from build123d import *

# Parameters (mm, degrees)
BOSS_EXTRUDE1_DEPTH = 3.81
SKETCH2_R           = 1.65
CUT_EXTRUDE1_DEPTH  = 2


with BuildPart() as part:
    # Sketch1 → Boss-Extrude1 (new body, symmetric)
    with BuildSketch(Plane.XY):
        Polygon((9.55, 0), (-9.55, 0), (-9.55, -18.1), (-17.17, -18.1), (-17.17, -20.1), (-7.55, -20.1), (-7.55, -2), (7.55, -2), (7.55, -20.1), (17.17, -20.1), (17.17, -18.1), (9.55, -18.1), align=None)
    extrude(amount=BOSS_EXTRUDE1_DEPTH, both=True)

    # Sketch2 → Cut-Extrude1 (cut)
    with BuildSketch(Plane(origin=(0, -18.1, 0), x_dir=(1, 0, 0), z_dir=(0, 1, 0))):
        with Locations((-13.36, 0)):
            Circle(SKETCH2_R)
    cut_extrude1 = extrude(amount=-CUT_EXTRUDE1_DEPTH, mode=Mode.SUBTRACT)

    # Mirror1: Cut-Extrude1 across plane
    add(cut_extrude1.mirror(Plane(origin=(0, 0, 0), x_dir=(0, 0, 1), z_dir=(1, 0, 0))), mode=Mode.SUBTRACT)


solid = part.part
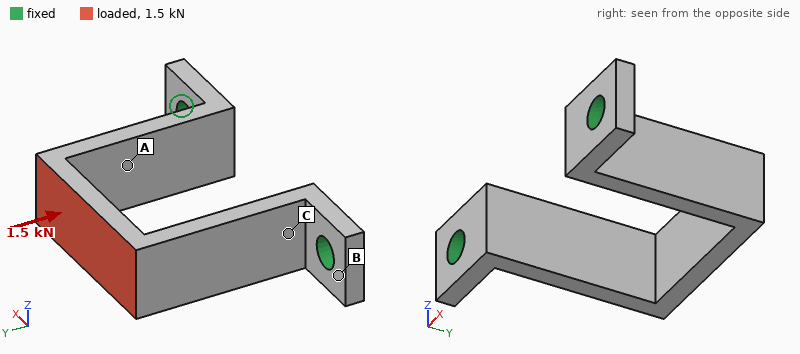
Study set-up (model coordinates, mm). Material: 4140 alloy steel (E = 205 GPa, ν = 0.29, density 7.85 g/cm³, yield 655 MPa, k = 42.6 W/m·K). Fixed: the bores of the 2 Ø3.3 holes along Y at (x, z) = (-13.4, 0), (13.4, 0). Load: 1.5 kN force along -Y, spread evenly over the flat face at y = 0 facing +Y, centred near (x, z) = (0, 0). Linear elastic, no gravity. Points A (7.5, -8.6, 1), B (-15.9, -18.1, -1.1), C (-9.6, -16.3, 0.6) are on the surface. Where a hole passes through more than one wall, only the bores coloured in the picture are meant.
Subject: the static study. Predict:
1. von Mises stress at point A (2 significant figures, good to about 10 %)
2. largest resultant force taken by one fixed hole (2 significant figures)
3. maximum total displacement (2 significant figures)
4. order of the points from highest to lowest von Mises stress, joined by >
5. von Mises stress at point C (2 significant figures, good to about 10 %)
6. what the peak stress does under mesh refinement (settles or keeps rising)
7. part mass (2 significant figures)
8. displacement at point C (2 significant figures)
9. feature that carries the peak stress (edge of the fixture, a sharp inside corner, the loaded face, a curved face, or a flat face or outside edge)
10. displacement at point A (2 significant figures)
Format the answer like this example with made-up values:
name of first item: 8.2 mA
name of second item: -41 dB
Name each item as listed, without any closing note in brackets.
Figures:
von Mises stress at point A: 120 MPa
largest resultant force taken by one fixed hole: 760 N
maximum total displacement: 48 µm
order of the points from highest to lowest von Mises stress, joined by >: C > A > B
von Mises stress at point C: 180 MPa
what the peak stress does under mesh refinement: keeps rising
part mass: 8.2 g
displacement at point C: 8.7 µm
feature that carries the peak stress: edge of the fixture
displacement at point A: 12 µm
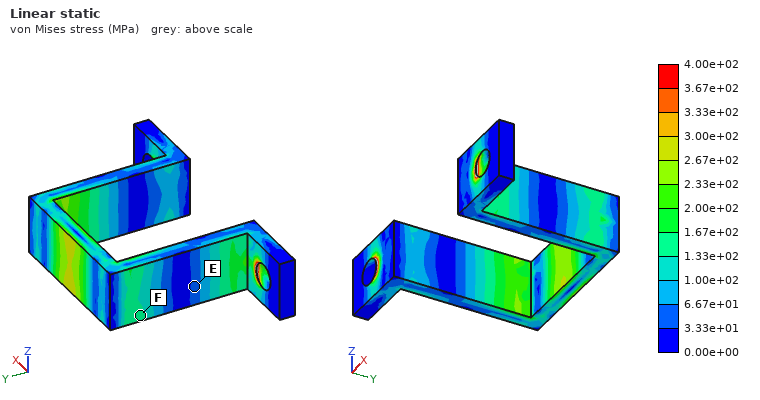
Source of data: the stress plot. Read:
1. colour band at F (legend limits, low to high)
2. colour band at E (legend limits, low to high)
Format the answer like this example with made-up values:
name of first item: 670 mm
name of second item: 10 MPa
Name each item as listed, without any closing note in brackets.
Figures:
colour band at F: 1.33e+02 to 1.67e+02 MPa
colour band at E: 3.33e+01 to 6.67e+01 MPa
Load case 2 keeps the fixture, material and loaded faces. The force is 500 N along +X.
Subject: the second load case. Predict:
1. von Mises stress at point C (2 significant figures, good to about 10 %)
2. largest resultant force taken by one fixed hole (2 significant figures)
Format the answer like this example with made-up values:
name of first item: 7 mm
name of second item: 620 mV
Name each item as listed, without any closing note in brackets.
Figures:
von Mises stress at point C: 310 MPa
largest resultant force taken by one fixed hole: 390 N
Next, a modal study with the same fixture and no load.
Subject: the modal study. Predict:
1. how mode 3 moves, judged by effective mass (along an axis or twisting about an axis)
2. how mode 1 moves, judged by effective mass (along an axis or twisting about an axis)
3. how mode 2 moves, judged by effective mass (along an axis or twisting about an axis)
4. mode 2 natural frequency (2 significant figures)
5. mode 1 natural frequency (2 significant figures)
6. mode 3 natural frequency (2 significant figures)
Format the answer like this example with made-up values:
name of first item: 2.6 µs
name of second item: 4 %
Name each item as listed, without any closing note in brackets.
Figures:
how mode 3 moves, judged by effective mass: twisting about Y
how mode 1 moves, judged by effective mass: along X
how mode 2 moves, judged by effective mass: along Z
mode 2 natural frequency: 4600 Hz
mode 1 natural frequency: 4200 Hz
mode 3 natural frequency: 7900 Hz
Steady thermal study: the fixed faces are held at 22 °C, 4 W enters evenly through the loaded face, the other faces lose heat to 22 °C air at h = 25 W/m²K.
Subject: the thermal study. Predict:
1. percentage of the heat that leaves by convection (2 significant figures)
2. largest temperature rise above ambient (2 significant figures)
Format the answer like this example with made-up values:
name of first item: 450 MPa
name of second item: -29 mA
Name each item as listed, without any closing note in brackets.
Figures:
percentage of the heat that leaves by convection: 21 %
largest temperature rise above ambient: 64 K
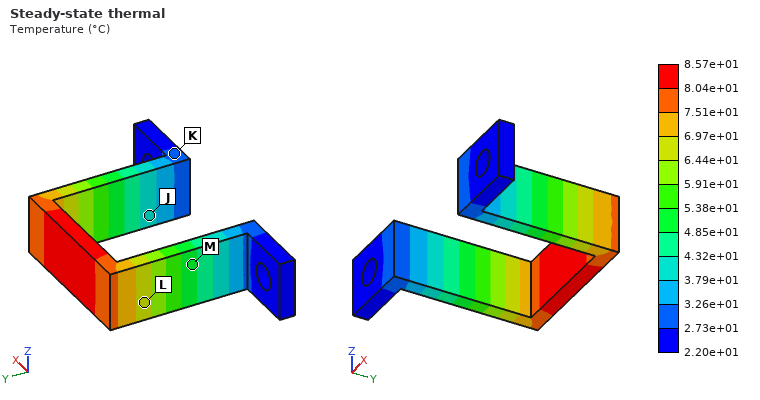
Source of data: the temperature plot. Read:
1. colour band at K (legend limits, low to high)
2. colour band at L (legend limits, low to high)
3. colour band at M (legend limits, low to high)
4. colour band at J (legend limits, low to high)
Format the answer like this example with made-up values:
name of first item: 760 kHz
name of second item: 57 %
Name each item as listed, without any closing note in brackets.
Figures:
colour band at K: 2.73e+01 to 3.26e+01 °C
colour band at L: 6.44e+01 to 6.97e+01 °C
colour band at M: 4.85e+01 to 5.38e+01 °C
colour band at J: 3.79e+01 to 4.32e+01 °C
